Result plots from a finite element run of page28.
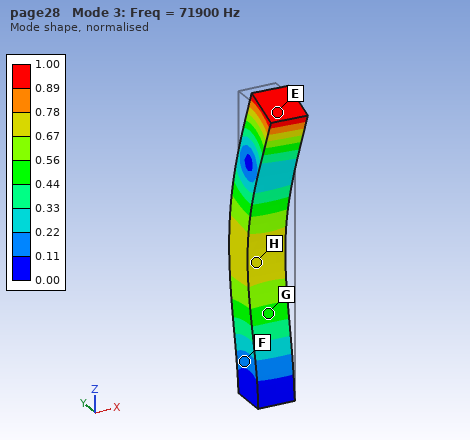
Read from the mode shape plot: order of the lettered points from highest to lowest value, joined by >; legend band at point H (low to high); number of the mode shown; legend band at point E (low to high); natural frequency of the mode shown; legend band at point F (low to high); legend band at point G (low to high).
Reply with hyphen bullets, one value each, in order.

- E > H > G > F
- 0.67 to 0.78
- 3
- 0.89 to 1.00
- 71900 Hz
- 0.11 to 0.22
- 0.44 to 0.56
